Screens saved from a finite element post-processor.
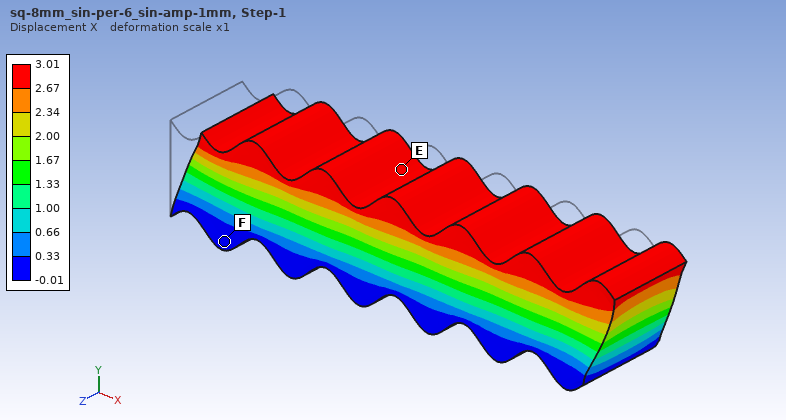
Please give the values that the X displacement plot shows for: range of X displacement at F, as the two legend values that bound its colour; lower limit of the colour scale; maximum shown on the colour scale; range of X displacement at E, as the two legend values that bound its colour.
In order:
-0.01 to 0.33
-0.01
3.01
2.67 to 3.01
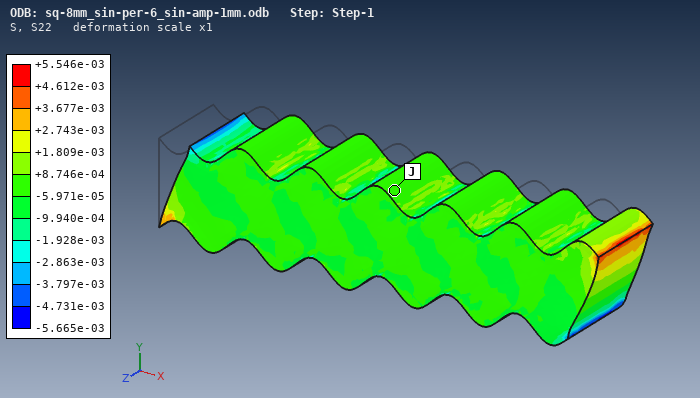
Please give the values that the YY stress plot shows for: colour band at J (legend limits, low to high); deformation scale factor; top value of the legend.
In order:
-5.971e-05 to +8.746e-04
1
+5.546e-03
